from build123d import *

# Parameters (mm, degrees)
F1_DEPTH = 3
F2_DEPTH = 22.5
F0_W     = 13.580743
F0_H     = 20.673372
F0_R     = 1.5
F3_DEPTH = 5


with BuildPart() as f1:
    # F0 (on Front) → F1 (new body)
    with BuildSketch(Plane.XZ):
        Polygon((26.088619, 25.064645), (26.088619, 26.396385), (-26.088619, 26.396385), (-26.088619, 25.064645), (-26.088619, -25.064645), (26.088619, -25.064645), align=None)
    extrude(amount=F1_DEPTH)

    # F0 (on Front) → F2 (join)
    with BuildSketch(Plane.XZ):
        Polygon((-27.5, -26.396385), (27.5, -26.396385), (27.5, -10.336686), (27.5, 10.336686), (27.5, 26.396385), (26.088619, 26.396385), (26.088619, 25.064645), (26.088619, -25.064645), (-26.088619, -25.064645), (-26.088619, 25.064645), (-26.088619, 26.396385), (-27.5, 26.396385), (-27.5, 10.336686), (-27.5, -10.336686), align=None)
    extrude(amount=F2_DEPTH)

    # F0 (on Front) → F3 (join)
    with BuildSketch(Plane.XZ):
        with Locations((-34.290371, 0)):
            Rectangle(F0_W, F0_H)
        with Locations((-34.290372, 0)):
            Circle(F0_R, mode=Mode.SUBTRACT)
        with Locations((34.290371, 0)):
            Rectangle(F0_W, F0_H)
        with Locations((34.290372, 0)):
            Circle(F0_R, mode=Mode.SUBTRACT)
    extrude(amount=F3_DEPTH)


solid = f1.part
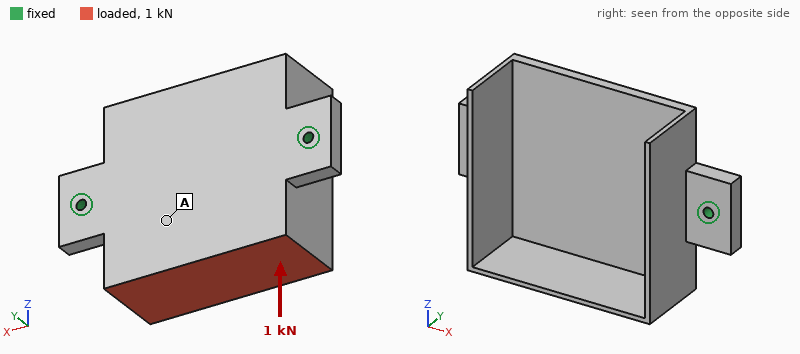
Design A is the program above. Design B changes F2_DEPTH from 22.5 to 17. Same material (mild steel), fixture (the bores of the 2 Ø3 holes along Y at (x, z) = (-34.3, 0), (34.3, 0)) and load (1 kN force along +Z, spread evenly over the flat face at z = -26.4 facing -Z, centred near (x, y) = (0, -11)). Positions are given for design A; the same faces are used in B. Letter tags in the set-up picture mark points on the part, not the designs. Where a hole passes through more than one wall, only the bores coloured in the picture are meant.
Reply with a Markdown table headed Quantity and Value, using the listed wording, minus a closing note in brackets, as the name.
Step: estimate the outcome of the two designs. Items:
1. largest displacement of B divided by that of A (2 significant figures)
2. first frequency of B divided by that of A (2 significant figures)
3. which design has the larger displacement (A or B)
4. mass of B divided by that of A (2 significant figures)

| Quantity | Value |
|---|---|
| largest displacement of B divided by that of A | 0.56 |
| first frequency of B divided by that of A | 1.1 |
| which design has the larger displacement | A |
| mass of B divided by that of A | 0.92 |
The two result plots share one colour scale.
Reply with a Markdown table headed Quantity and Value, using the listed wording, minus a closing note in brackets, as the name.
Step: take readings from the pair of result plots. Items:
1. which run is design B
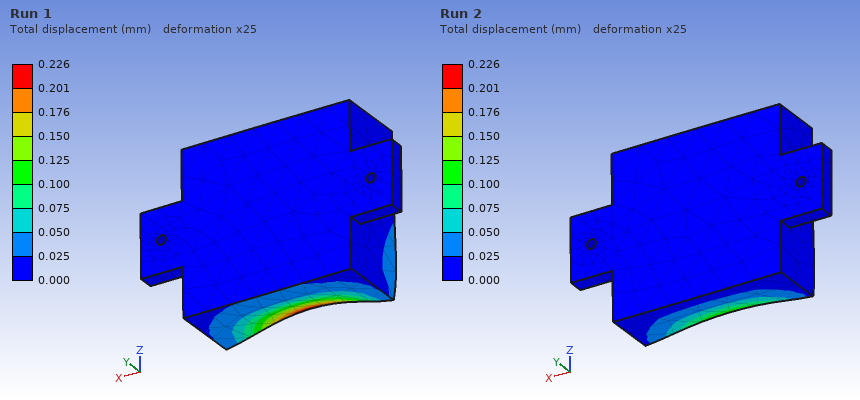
| Quantity | Value |
|---|---|
| which run is design B | Run 2 |
